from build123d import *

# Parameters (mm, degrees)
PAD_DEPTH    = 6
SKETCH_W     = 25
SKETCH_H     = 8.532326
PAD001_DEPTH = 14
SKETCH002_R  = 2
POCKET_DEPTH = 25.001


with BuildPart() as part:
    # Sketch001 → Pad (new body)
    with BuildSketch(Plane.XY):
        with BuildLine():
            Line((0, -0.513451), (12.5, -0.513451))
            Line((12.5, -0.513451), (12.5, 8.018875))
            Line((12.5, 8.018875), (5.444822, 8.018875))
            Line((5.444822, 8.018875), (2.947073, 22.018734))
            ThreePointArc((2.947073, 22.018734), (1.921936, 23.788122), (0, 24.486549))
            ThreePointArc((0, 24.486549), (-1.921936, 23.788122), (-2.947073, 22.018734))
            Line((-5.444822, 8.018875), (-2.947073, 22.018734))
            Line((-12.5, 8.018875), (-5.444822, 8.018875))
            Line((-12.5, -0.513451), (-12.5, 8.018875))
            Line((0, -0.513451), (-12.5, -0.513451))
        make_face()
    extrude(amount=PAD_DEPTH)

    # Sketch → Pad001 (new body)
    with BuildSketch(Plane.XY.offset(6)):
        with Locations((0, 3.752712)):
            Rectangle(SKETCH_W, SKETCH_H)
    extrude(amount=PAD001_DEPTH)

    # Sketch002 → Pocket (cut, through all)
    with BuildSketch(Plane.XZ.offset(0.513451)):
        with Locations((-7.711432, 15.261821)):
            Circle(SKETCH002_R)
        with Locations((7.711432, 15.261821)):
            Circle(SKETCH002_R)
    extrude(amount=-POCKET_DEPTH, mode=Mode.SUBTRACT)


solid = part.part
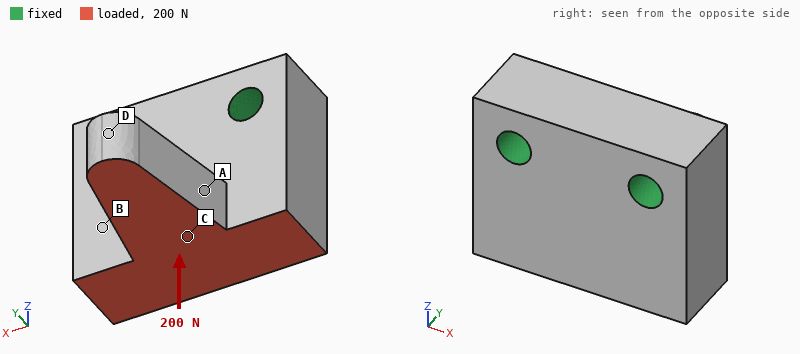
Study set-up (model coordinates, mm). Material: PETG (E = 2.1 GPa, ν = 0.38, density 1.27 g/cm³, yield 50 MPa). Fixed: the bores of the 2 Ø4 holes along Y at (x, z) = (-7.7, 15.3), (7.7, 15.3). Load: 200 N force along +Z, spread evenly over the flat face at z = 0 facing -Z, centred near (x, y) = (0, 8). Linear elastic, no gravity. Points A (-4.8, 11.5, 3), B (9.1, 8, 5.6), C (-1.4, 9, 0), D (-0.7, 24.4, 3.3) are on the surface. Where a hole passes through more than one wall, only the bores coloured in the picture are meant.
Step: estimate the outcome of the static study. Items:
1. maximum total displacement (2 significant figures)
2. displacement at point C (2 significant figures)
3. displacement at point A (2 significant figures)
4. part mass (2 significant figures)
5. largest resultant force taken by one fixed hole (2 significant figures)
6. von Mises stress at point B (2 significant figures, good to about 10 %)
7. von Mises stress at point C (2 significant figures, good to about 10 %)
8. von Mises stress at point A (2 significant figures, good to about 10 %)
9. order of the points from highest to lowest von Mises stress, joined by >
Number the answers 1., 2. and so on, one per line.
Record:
1. 0.26 mm
2. 0.066 mm
3. 0.064 mm
4. 6.1 g
5. 100 N
6. 2.2 MPa
7. 6.4 MPa
8. 3.5 MPa
9. C > A > B > D
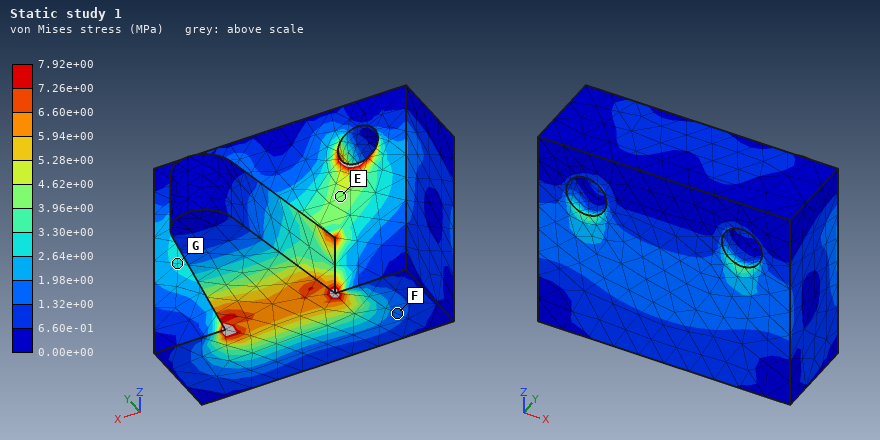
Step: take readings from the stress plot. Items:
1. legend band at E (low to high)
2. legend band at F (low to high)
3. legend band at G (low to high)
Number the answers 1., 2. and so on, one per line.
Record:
1. 3.96e+00 to 4.62e+00 MPa
2. 1.32e+00 to 1.98e+00 MPa
3. 2.64e+00 to 3.30e+00 MPa
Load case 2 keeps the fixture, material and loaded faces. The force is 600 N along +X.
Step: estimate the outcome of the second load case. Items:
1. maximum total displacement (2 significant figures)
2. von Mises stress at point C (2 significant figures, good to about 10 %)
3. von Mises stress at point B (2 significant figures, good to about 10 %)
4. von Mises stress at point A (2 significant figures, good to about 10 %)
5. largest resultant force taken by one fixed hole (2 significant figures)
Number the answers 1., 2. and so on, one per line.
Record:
1. 0.42 mm
2. 9.7 MPa
3. 6.1 MPa
4. 14 MPa
5. 590 N
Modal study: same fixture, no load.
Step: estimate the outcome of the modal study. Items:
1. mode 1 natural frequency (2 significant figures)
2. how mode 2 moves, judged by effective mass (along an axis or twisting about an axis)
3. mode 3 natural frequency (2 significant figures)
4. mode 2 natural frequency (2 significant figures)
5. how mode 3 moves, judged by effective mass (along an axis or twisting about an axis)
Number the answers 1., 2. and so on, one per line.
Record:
1. 3400 Hz
2. along X
3. 6200 Hz
4. 4900 Hz
5. along Y
